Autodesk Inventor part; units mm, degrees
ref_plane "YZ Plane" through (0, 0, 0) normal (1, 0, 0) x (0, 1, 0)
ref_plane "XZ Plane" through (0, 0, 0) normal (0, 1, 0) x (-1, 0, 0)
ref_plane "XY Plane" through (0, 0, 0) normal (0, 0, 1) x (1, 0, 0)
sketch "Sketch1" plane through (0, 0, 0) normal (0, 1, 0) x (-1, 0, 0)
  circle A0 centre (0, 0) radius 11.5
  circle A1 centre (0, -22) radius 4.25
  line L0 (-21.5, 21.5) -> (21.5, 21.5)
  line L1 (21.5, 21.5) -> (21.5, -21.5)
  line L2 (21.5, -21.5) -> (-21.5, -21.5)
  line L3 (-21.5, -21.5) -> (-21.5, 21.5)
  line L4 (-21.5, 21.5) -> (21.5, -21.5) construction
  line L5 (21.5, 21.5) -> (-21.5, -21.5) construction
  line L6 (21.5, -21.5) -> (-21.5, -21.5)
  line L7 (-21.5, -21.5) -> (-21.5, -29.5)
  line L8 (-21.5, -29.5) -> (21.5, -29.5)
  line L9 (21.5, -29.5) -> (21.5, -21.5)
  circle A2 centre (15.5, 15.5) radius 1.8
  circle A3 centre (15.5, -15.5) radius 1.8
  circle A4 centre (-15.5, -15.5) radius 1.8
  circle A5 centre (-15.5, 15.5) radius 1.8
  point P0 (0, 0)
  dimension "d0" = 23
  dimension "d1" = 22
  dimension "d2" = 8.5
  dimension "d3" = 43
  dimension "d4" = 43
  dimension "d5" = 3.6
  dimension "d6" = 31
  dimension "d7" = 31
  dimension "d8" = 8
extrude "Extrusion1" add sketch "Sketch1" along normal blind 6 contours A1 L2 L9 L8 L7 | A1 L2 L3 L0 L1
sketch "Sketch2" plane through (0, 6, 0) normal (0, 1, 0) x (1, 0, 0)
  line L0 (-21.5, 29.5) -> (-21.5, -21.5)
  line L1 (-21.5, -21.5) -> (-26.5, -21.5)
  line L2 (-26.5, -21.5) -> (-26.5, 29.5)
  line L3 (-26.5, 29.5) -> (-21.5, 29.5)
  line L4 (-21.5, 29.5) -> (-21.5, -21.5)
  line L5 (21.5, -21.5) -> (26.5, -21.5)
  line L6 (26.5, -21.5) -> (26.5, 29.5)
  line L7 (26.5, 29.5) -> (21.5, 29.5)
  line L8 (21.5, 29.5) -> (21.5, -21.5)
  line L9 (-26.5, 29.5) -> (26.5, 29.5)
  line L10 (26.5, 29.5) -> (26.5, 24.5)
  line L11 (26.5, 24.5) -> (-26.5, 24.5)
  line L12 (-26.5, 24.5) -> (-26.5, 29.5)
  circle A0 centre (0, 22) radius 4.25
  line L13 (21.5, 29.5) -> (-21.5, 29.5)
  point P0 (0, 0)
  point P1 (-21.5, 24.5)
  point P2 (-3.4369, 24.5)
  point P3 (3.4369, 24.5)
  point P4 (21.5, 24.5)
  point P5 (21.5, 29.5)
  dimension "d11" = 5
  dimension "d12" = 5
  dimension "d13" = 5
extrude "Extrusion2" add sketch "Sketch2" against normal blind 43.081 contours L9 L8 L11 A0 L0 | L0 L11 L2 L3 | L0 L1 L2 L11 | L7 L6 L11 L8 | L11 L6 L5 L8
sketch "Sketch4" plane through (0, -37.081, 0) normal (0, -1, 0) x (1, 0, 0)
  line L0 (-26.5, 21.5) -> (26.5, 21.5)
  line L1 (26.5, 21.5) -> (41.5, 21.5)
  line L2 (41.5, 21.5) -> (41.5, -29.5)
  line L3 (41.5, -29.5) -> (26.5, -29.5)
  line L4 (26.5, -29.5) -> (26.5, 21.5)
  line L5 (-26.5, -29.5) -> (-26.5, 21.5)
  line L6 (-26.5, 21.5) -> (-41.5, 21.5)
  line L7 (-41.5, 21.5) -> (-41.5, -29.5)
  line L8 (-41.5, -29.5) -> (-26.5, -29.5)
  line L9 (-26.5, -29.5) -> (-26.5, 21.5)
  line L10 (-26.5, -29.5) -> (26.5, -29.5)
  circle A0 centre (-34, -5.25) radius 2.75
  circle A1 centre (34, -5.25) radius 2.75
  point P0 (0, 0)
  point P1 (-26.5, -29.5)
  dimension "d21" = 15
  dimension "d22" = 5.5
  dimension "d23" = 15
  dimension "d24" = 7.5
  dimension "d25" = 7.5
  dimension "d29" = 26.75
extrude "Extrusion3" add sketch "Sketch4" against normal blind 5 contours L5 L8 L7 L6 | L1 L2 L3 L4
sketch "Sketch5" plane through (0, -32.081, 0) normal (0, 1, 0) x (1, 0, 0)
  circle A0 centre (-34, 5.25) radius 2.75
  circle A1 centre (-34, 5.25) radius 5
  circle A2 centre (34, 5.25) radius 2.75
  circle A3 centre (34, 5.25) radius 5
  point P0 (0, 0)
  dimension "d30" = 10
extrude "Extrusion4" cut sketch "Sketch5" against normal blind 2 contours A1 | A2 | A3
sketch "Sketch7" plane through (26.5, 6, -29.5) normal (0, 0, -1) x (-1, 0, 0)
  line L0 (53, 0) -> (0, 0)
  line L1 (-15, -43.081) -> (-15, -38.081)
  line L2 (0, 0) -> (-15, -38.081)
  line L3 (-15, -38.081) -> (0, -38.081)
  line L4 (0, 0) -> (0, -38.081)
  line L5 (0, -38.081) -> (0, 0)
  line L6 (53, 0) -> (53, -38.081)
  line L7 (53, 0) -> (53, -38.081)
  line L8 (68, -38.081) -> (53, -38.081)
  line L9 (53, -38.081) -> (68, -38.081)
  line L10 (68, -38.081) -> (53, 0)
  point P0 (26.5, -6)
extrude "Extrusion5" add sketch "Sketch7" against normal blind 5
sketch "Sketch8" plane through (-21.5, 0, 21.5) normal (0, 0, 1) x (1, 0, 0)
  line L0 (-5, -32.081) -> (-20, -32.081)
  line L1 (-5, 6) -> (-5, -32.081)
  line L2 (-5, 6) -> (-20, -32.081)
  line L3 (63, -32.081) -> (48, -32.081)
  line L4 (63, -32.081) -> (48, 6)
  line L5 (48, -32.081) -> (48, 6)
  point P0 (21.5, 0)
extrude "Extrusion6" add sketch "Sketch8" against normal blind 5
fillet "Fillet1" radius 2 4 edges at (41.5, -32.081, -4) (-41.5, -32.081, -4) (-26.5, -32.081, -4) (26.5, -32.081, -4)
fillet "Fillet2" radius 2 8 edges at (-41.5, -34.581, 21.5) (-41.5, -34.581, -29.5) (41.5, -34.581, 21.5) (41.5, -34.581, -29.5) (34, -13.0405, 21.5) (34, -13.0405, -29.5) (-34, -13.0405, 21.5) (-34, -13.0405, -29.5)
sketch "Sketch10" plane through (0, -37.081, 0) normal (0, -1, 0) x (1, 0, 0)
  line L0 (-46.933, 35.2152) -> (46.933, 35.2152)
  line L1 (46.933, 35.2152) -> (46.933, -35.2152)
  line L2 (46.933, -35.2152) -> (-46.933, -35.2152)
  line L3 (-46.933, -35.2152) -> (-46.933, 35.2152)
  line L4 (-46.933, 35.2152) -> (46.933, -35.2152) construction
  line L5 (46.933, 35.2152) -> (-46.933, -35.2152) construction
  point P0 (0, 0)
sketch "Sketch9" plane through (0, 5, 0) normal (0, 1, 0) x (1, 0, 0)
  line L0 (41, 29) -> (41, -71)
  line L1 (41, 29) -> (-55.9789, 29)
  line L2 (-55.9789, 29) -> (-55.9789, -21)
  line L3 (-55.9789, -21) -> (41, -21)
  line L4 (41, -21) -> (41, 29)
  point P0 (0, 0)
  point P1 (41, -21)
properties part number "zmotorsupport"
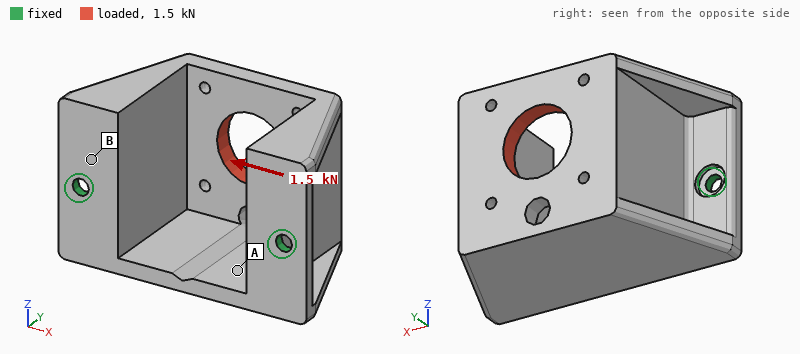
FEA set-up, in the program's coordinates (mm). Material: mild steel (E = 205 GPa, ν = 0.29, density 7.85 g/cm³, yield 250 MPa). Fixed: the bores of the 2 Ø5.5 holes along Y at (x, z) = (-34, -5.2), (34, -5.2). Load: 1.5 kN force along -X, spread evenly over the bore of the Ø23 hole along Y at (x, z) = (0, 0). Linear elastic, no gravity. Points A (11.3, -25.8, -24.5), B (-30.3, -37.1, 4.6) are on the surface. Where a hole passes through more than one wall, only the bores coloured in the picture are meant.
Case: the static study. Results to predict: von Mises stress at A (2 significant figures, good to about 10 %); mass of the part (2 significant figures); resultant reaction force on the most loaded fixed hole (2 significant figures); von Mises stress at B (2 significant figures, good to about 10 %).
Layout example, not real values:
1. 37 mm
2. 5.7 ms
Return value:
1. 16 MPa
2. 410 g
3. 1.1 kN
4. 26 MPa
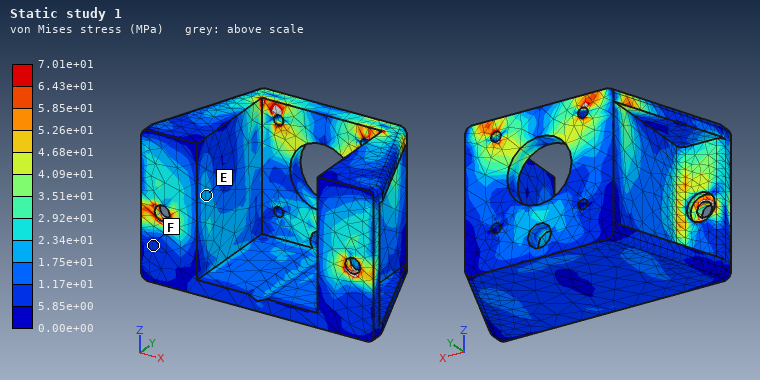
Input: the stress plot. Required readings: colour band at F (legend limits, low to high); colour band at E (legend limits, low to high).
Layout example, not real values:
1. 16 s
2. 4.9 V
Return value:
1. 5.85e+00 to 1.17e+01 MPa
2. 1.75e+01 to 2.34e+01 MPa
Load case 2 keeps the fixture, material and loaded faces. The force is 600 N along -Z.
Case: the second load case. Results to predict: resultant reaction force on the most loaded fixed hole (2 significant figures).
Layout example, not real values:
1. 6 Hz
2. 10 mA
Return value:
1. 350 N
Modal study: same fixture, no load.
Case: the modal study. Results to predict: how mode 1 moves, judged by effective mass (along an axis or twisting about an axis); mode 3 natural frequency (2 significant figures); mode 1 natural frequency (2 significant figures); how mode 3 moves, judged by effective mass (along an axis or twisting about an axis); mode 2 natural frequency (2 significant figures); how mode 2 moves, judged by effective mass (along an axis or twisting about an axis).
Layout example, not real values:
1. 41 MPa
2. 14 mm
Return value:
1. along Z
2. 4500 Hz
3. 990 Hz
4. along X
5. 2300 Hz
6. along X
